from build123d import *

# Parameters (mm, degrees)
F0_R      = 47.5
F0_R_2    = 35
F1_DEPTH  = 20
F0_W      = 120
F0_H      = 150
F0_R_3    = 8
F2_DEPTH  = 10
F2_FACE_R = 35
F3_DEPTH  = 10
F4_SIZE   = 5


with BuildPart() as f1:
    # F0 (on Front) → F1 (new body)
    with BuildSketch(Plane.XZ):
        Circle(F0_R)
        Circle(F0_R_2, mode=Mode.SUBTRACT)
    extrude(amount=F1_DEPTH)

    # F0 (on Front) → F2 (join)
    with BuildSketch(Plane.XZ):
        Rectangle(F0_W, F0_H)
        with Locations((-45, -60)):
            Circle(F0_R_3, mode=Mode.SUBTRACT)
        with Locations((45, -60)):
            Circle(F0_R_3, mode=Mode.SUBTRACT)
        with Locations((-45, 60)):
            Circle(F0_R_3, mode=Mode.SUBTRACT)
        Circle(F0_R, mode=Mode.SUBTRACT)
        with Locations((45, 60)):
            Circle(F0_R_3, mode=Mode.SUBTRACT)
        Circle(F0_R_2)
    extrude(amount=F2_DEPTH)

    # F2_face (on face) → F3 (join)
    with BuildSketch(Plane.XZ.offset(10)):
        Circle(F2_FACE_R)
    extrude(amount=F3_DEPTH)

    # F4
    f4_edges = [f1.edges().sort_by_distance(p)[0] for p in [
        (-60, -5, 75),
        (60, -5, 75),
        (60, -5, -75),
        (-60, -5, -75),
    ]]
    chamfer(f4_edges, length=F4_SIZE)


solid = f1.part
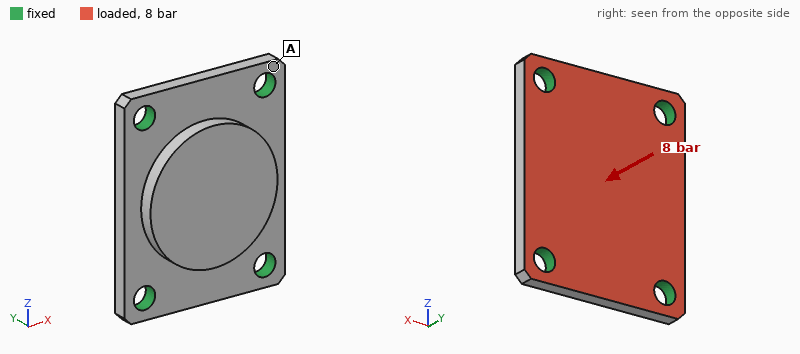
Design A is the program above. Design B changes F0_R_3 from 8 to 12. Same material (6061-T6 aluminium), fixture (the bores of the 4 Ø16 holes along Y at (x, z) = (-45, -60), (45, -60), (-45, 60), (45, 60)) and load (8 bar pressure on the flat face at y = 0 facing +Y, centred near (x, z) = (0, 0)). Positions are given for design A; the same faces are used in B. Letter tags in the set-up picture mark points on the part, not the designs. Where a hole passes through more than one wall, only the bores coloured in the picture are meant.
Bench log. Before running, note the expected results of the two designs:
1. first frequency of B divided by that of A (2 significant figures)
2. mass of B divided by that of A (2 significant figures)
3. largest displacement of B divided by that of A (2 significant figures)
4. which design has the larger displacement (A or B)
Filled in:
1.2
0.96
0.70
A
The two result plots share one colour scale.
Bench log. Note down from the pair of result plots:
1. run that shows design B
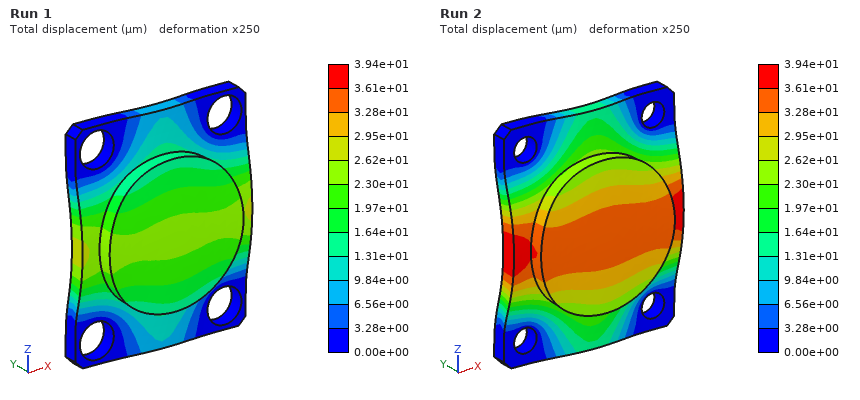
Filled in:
Run 1
